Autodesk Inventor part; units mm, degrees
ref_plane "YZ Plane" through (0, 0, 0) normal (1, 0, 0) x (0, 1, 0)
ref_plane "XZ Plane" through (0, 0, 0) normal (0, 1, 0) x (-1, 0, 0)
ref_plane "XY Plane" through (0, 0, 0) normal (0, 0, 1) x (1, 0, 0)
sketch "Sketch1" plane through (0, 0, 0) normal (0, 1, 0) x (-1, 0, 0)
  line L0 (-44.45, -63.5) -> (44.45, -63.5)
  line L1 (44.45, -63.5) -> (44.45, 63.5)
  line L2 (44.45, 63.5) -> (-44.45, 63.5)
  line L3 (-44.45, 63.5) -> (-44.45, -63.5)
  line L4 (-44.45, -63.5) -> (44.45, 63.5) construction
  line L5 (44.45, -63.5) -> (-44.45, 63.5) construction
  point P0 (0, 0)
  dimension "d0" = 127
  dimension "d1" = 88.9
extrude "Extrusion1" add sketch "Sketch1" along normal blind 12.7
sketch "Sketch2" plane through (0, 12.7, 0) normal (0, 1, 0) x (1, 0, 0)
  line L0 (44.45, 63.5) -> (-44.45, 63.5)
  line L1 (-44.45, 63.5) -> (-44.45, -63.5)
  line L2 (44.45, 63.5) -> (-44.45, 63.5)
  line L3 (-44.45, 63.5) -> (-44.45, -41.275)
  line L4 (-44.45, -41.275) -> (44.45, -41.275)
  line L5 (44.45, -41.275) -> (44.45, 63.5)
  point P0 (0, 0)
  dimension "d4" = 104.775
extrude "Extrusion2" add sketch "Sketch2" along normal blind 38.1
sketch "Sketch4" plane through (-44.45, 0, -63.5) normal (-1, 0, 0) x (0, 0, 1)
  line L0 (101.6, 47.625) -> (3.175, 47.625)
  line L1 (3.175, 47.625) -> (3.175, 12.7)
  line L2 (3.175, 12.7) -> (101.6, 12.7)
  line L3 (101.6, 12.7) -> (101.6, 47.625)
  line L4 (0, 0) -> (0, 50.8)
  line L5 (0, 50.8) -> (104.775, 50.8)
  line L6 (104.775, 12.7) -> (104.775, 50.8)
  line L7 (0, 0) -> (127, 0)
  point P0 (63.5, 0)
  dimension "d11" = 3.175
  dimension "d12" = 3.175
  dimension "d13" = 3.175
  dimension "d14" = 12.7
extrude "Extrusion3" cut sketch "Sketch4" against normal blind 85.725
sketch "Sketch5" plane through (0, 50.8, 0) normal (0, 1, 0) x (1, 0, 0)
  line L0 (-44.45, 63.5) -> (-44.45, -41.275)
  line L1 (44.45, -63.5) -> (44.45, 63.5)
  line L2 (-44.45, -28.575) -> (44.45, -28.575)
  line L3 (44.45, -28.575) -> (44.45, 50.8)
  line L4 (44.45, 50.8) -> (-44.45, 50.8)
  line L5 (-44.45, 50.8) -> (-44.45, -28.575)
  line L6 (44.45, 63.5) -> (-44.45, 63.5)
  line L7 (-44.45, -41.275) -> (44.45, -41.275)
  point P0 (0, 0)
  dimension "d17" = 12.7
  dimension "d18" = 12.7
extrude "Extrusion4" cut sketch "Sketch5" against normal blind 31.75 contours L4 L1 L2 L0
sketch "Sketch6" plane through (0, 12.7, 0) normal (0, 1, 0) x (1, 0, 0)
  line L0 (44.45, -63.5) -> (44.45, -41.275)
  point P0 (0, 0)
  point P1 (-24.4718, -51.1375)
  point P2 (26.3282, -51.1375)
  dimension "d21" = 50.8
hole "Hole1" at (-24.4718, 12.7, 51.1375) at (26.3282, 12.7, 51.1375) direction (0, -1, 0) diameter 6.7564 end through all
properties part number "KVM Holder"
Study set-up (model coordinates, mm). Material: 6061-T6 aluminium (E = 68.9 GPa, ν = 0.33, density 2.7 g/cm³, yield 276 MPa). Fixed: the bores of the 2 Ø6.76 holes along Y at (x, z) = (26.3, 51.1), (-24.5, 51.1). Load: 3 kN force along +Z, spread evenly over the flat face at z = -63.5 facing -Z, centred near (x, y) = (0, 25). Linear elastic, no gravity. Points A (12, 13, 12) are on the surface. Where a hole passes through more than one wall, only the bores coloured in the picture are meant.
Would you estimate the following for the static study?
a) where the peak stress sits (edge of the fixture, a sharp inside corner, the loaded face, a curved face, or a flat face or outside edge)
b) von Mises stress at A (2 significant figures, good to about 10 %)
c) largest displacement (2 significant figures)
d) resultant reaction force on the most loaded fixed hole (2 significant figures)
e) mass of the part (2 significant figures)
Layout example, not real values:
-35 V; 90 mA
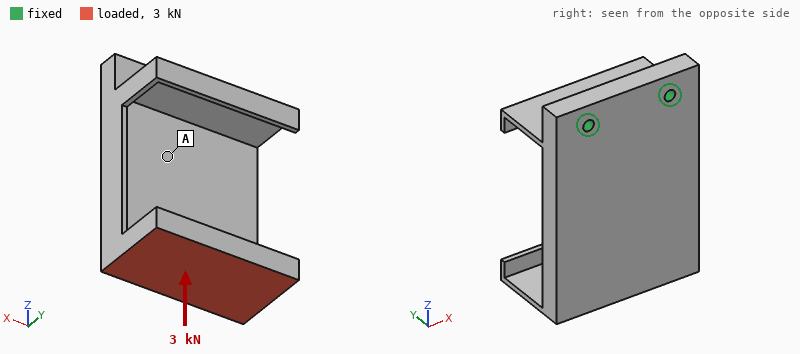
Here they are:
the loaded face; 22 MPa; 1.2 mm; 1.6 kN; 470 g
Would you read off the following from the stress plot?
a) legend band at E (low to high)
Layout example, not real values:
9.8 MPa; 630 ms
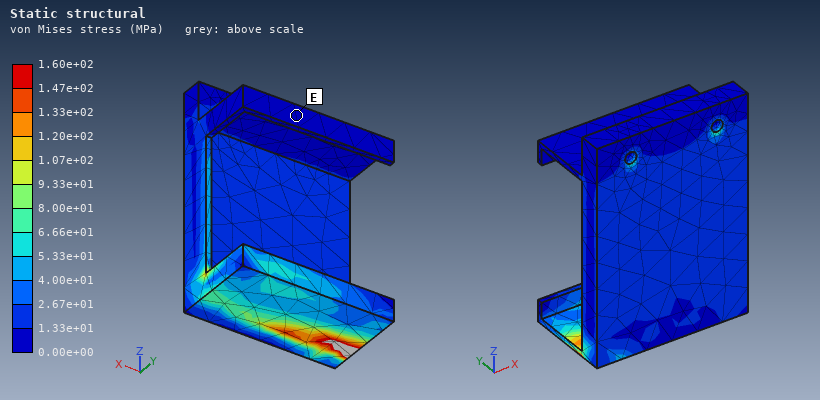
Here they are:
0.00e+00 to 1.33e+01 MPa
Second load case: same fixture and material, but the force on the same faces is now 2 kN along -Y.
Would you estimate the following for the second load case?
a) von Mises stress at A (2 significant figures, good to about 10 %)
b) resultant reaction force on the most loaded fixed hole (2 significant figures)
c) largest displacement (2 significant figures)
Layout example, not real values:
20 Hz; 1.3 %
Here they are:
51 MPa; 1.1 kN; 1.2 mm
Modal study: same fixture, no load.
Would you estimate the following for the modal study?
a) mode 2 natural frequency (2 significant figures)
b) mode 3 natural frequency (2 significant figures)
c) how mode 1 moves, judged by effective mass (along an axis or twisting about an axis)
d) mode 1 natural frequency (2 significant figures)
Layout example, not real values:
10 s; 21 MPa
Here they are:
1500 Hz; 1500 Hz; along Y; 630 Hz
